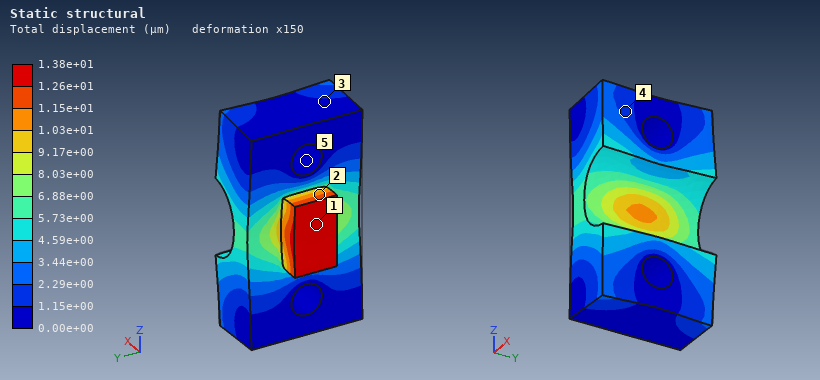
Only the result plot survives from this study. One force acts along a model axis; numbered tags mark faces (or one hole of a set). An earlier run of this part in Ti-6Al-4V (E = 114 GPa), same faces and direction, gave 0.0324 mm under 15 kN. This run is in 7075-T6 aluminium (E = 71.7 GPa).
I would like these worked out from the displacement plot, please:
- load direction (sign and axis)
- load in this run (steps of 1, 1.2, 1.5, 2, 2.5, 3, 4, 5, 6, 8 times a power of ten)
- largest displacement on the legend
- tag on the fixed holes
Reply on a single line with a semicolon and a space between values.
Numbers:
+X; 4 kN; 1.38e+01 µm; 5
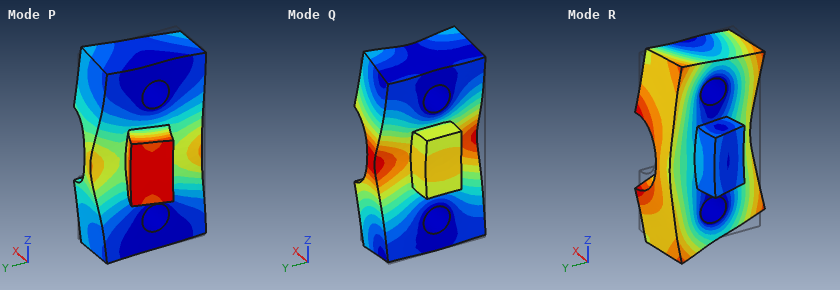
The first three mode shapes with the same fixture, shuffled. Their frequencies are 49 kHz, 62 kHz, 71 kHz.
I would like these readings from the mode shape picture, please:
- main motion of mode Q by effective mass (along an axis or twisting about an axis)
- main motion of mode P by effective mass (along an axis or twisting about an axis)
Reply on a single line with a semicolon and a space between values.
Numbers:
along X; along Y
